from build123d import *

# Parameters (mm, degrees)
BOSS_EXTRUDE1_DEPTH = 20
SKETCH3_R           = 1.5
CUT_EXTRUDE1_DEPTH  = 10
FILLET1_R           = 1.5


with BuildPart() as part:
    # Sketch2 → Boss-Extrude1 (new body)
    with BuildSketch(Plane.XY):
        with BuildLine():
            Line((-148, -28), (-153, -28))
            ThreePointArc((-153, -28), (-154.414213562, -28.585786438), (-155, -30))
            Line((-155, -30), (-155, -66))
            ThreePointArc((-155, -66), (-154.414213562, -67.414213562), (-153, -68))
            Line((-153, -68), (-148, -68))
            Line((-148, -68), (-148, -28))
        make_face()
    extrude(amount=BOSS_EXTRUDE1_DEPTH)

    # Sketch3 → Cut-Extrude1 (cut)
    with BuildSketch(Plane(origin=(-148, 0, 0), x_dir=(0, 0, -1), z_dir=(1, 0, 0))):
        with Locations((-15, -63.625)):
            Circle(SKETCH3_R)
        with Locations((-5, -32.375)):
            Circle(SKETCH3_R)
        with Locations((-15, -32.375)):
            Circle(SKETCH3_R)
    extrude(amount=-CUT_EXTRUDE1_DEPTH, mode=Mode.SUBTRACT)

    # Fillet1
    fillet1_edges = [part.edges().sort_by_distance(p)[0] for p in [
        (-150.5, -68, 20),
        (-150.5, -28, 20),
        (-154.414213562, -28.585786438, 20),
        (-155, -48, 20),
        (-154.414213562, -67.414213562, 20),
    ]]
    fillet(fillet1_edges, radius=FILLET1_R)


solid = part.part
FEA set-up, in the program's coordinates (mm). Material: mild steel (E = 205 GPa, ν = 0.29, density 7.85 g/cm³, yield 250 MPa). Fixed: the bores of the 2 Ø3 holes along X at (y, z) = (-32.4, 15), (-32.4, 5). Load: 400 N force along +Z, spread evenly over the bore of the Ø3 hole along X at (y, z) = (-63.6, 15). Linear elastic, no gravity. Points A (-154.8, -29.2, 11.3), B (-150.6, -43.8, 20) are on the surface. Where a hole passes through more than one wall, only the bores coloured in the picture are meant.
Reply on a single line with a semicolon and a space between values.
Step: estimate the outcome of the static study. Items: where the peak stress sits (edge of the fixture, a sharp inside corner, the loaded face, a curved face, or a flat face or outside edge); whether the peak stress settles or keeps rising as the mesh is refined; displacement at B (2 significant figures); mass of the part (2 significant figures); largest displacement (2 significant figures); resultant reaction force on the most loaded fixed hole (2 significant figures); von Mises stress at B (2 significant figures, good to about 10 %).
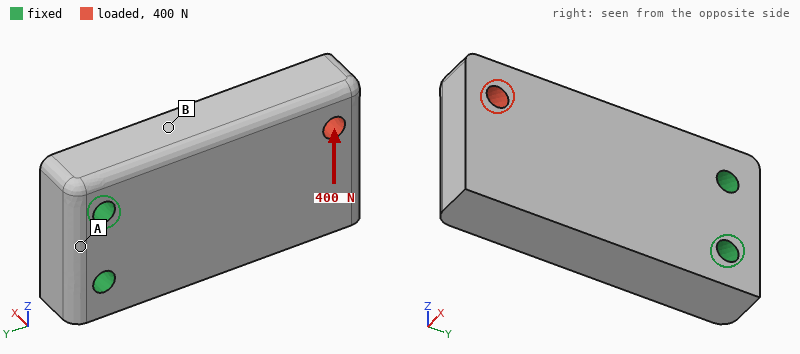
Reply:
edge of the fixture; keeps rising; 2.2 µm; 42 g; 7.8 µm; 1.0 kN; 17 MPa
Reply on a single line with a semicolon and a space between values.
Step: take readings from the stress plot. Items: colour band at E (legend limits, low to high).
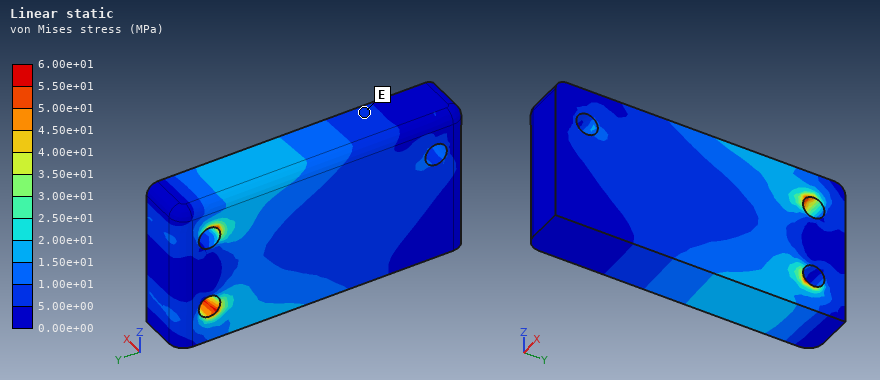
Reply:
5.00e+00 to 1.00e+01 MPa
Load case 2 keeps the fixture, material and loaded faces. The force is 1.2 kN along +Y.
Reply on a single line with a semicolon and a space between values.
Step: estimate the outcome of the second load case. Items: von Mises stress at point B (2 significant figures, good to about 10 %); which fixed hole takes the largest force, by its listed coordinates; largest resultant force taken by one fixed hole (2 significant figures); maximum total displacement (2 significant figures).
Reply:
21 MPa; (-32.4, 15); 1.1 kN; 5.1 µm
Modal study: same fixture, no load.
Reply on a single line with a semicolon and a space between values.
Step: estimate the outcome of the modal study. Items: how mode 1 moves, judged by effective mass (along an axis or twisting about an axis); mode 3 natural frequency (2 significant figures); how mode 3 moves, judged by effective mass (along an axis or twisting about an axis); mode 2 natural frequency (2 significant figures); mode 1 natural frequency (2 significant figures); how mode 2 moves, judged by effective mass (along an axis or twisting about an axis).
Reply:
along X; 15 kHz; twisting about Y; 10 kHz; 4500 Hz; along Z
